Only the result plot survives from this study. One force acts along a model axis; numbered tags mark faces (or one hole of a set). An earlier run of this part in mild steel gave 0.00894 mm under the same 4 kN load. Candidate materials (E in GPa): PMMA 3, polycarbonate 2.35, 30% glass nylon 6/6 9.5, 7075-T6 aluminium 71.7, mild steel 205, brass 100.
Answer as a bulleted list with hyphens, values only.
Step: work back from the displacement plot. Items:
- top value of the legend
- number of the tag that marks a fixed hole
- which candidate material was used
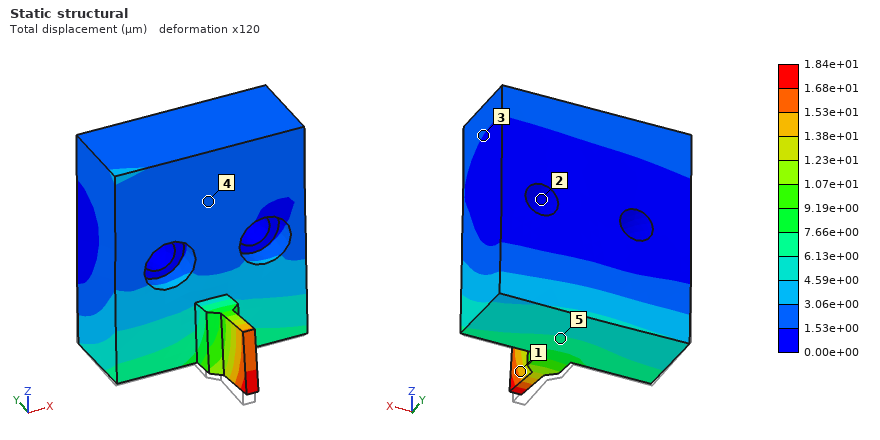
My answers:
- 1.84e+01 µm
- 2
- brass
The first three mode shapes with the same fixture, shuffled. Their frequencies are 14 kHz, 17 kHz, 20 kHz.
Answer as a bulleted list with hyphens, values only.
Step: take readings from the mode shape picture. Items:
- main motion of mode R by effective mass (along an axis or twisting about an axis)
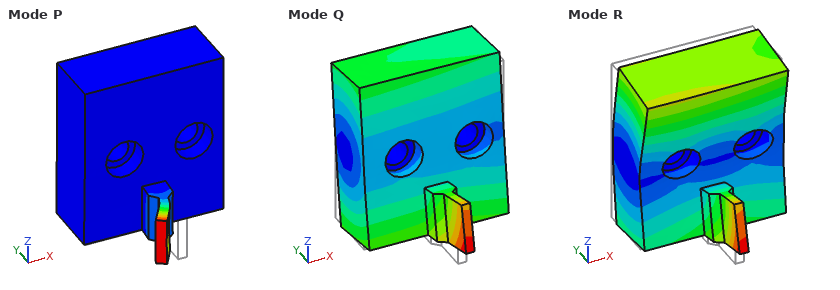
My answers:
- along Y
